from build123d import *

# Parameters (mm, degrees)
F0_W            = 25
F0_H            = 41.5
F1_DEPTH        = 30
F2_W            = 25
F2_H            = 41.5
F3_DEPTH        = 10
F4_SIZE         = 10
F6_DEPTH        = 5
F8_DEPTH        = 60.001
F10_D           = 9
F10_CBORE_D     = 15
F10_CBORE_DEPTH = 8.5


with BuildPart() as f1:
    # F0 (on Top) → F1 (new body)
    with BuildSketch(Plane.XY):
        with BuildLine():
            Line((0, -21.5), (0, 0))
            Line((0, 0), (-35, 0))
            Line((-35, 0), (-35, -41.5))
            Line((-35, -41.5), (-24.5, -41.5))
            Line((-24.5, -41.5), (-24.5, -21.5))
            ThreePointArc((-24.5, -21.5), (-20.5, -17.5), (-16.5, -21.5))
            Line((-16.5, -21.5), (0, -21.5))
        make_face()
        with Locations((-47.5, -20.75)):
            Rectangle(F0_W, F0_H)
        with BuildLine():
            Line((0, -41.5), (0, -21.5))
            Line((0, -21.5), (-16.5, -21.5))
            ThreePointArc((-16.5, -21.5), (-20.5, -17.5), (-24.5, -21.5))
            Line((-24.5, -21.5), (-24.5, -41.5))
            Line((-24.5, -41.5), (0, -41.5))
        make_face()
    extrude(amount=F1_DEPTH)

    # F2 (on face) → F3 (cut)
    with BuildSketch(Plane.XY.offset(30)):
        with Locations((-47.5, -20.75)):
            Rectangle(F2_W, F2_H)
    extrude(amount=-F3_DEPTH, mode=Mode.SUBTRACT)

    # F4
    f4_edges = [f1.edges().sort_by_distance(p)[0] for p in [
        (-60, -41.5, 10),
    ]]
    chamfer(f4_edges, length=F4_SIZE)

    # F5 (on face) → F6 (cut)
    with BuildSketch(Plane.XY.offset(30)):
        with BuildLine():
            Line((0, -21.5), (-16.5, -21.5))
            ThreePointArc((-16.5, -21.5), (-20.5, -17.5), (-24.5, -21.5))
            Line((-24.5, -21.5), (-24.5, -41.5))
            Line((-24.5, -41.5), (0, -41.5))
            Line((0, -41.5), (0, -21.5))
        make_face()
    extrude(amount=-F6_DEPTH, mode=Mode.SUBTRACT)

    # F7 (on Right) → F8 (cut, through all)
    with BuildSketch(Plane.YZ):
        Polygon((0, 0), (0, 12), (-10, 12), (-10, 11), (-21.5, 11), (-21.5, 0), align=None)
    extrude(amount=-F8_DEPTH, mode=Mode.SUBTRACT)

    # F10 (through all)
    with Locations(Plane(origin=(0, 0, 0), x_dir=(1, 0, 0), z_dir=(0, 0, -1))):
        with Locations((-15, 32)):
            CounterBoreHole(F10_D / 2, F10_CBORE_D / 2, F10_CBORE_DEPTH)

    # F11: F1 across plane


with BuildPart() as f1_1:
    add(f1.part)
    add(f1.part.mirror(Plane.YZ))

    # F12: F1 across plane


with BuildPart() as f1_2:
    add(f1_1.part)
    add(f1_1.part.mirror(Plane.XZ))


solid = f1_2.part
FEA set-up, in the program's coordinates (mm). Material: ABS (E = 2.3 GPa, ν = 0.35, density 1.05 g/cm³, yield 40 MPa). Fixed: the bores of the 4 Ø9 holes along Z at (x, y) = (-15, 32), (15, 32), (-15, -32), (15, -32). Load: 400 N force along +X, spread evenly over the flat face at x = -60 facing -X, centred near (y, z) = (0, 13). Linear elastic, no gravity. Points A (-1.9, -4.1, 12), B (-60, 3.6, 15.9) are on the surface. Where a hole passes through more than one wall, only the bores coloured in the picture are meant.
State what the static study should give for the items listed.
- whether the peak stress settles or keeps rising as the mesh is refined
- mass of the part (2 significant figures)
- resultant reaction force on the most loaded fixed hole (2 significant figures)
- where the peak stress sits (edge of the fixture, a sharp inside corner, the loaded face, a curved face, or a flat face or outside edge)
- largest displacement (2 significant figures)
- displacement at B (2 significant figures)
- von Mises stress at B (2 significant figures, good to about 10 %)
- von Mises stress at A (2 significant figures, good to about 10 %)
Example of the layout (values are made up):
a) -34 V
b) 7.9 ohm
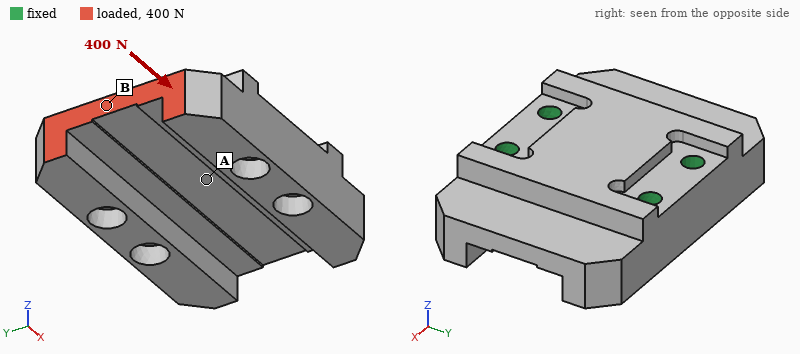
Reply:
a) keeps rising
b) 180 g
c) 160 N
d) edge of the fixture
e) 17 µm
f) 13 µm
g) 0.46 MPa
h) 0.16 MPa
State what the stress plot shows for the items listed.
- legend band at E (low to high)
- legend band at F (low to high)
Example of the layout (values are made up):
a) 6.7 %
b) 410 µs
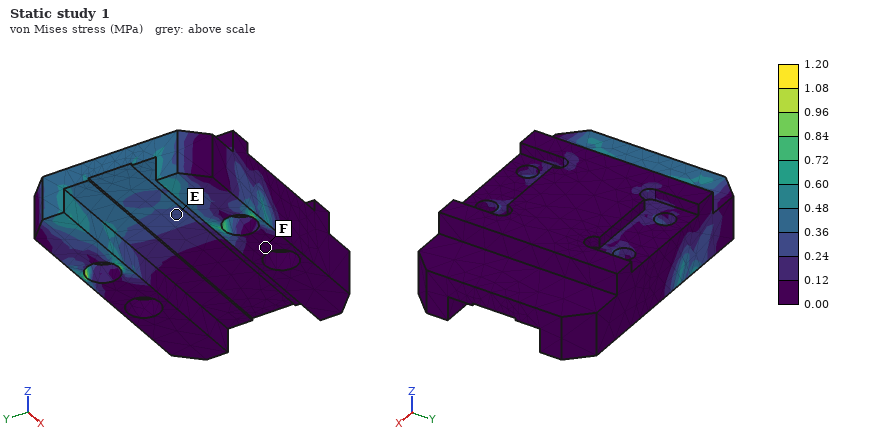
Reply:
a) 0.24 to 0.36 MPa
b) 0.00 to 0.12 MPa
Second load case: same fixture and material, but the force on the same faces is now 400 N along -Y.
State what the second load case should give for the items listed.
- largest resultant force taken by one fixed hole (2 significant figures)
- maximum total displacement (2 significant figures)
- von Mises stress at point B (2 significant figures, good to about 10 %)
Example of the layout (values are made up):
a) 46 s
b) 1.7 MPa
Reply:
a) 300 N
b) 49 µm
c) 0.95 MPa
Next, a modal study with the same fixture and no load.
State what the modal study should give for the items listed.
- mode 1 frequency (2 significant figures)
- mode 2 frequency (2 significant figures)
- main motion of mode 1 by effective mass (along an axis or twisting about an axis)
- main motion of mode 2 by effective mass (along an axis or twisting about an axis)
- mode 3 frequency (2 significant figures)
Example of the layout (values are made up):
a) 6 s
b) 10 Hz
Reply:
a) 2000 Hz
b) 2100 Hz
c) twisting about Y
d) along Z
e) 2600 Hz
